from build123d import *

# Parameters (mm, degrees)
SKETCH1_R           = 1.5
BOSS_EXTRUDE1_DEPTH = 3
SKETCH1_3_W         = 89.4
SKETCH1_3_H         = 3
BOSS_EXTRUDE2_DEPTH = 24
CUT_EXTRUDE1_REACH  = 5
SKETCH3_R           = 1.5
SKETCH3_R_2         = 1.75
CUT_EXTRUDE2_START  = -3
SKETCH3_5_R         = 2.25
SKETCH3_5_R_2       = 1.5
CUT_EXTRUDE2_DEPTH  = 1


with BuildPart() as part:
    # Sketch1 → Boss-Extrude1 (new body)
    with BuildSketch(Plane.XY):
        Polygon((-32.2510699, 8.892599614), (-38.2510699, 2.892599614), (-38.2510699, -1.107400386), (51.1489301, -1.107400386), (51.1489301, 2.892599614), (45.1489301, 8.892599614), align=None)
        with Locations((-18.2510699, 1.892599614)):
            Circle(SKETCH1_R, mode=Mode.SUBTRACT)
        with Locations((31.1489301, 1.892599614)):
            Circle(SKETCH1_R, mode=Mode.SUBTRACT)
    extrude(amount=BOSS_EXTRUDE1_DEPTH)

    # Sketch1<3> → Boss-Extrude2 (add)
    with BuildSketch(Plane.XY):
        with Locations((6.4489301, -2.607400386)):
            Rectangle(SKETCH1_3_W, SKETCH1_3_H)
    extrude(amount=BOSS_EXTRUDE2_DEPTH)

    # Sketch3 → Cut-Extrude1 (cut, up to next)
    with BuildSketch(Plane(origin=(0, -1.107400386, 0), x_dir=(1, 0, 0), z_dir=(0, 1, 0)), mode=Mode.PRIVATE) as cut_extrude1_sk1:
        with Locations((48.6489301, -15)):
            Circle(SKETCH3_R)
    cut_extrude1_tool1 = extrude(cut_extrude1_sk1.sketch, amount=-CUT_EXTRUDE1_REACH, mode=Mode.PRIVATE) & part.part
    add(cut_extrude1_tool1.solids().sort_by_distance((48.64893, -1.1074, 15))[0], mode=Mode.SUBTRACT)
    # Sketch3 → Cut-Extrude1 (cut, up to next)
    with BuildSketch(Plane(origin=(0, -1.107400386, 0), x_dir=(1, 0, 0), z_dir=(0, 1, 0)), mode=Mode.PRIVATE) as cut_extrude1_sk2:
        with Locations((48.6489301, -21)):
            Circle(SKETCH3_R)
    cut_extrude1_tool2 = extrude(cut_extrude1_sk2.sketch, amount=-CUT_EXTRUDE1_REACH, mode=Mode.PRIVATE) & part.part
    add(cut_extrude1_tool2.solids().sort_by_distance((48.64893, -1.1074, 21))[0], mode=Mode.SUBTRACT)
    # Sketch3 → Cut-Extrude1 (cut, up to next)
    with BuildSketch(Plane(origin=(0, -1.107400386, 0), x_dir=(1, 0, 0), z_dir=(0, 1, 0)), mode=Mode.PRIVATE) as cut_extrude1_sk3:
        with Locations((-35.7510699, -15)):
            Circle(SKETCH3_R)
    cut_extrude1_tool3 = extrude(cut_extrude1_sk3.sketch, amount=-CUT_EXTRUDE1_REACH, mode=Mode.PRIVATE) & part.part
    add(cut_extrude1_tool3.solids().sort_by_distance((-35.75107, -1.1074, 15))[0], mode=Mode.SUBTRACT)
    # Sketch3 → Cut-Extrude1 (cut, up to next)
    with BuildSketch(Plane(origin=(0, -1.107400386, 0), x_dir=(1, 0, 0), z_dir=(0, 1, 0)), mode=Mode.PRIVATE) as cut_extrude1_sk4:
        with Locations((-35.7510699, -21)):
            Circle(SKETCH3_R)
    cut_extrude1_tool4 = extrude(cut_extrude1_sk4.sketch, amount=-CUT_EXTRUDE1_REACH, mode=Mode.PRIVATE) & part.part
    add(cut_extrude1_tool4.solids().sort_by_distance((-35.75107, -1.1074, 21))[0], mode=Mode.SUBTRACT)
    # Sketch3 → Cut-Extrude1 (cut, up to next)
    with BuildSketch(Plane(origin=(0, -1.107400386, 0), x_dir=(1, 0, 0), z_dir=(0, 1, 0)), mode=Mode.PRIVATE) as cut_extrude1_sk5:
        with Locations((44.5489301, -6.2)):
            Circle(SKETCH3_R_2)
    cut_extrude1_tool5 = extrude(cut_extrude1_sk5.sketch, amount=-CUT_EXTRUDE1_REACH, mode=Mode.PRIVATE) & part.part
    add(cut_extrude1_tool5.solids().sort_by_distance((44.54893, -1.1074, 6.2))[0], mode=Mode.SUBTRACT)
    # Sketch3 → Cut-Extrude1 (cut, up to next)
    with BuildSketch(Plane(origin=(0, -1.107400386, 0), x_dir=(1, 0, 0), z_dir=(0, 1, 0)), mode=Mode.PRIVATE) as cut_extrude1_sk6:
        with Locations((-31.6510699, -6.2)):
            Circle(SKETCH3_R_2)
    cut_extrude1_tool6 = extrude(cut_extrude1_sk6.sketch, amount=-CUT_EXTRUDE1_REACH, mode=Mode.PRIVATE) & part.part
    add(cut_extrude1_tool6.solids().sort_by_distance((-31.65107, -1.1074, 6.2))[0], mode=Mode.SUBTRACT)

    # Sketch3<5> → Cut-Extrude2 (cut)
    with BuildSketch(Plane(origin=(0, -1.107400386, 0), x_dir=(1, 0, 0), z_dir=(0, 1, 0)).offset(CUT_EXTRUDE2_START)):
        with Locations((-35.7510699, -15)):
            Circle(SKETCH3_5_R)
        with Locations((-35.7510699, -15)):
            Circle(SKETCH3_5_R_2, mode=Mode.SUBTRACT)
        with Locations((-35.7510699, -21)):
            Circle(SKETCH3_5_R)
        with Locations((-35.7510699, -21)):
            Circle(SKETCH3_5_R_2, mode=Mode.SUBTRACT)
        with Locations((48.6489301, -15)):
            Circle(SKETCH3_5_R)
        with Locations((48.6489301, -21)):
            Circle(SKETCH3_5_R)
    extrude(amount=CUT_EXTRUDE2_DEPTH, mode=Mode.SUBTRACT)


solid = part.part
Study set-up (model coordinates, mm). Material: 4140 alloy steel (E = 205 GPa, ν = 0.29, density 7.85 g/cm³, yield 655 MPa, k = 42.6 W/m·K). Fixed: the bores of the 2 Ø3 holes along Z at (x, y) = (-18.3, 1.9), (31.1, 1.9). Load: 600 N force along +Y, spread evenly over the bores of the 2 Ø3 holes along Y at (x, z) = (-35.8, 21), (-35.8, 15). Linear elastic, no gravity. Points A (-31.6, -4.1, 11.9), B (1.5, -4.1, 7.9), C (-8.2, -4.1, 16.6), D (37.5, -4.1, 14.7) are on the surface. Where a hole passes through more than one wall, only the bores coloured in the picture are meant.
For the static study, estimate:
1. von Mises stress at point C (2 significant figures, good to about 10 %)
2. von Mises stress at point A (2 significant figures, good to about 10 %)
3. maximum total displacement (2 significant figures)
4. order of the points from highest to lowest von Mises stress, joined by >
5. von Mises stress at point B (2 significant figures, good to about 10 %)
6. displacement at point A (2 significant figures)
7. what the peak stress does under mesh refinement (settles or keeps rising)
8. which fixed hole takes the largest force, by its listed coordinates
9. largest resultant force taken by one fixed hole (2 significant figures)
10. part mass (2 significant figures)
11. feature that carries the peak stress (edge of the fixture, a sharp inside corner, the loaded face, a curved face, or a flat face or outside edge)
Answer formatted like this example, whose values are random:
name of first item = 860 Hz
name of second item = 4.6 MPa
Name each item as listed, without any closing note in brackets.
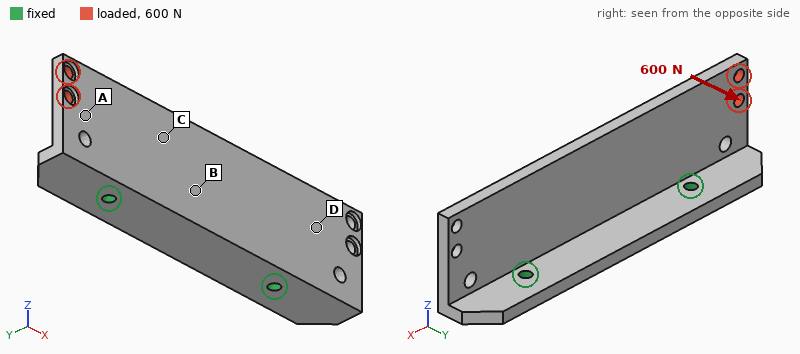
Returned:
von Mises stress at point C = 92 MPa
von Mises stress at point A = 160 MPa
maximum total displacement = 0.31 mm
order of the points from highest to lowest von Mises stress, joined by > = A > C > B > D
von Mises stress at point B = 49 MPa
displacement at point A = 0.12 mm
what the peak stress does under mesh refinement = keeps rising
which fixed hole takes the largest force, by its listed coordinates = (-18.3, 1.9)
largest resultant force taken by one fixed hole = 760 N
part mass = 69 g
feature that carries the peak stress = edge of the fixture
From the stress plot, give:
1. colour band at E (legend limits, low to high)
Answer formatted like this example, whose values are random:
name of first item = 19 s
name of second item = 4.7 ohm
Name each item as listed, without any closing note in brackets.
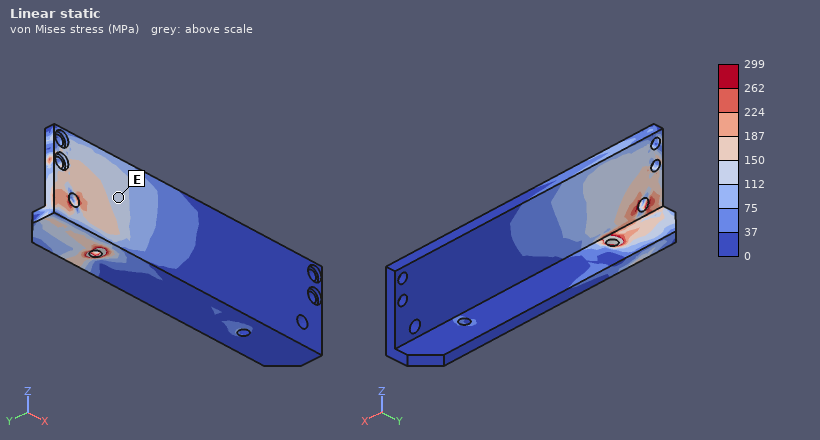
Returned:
colour band at E = 112 to 150 MPa
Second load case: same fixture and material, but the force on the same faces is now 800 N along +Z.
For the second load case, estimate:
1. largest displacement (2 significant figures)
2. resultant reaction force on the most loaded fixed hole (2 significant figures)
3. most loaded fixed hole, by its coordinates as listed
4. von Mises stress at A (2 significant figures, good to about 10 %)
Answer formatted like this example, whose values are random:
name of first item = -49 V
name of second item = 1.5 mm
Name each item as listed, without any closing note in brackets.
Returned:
largest displacement = 29 µm
resultant reaction force on the most loaded fixed hole = 1.1 kN
most loaded fixed hole, by its coordinates as listed = (-18.3, 1.9)
von Mises stress at A = 27 MPa
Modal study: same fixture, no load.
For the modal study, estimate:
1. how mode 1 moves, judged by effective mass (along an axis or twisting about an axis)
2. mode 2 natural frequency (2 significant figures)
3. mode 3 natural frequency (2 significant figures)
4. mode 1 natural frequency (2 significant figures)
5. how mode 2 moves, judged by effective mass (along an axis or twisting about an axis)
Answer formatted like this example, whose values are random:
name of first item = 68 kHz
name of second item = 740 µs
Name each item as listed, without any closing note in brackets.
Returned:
how mode 1 moves, judged by effective mass = along Y
mode 2 natural frequency = 4000 Hz
mode 3 natural frequency = 5600 Hz
mode 1 natural frequency = 2900 Hz
how mode 2 moves, judged by effective mass = twisting about Z
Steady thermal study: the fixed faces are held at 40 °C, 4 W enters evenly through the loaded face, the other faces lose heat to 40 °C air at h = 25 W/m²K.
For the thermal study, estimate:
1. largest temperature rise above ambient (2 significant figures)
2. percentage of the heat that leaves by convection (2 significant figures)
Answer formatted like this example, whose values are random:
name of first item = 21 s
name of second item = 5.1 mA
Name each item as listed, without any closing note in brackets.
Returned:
largest temperature rise above ambient = 45 K
percentage of the heat that leaves by convection = 25 %
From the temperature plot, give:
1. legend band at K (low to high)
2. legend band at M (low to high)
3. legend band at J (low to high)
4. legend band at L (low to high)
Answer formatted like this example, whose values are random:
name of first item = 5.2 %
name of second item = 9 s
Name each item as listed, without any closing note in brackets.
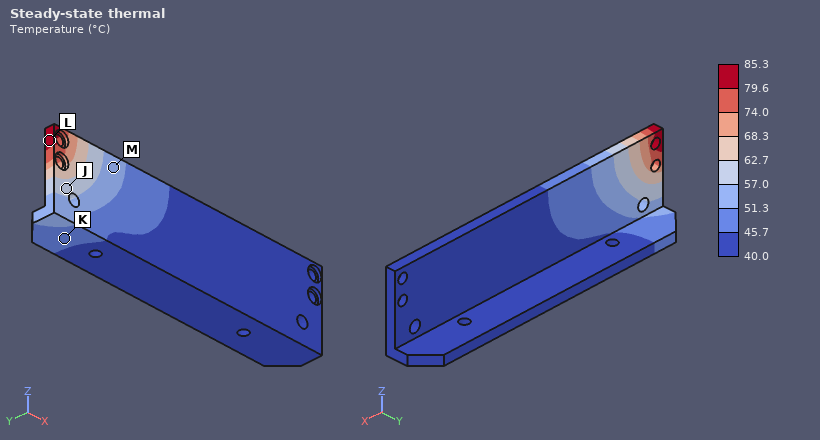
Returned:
legend band at K = 45.7 to 51.3 °C
legend band at M = 51.3 to 57.0 °C
legend band at J = 57.0 to 62.7 °C
legend band at L = 79.6 to 85.3 °C
